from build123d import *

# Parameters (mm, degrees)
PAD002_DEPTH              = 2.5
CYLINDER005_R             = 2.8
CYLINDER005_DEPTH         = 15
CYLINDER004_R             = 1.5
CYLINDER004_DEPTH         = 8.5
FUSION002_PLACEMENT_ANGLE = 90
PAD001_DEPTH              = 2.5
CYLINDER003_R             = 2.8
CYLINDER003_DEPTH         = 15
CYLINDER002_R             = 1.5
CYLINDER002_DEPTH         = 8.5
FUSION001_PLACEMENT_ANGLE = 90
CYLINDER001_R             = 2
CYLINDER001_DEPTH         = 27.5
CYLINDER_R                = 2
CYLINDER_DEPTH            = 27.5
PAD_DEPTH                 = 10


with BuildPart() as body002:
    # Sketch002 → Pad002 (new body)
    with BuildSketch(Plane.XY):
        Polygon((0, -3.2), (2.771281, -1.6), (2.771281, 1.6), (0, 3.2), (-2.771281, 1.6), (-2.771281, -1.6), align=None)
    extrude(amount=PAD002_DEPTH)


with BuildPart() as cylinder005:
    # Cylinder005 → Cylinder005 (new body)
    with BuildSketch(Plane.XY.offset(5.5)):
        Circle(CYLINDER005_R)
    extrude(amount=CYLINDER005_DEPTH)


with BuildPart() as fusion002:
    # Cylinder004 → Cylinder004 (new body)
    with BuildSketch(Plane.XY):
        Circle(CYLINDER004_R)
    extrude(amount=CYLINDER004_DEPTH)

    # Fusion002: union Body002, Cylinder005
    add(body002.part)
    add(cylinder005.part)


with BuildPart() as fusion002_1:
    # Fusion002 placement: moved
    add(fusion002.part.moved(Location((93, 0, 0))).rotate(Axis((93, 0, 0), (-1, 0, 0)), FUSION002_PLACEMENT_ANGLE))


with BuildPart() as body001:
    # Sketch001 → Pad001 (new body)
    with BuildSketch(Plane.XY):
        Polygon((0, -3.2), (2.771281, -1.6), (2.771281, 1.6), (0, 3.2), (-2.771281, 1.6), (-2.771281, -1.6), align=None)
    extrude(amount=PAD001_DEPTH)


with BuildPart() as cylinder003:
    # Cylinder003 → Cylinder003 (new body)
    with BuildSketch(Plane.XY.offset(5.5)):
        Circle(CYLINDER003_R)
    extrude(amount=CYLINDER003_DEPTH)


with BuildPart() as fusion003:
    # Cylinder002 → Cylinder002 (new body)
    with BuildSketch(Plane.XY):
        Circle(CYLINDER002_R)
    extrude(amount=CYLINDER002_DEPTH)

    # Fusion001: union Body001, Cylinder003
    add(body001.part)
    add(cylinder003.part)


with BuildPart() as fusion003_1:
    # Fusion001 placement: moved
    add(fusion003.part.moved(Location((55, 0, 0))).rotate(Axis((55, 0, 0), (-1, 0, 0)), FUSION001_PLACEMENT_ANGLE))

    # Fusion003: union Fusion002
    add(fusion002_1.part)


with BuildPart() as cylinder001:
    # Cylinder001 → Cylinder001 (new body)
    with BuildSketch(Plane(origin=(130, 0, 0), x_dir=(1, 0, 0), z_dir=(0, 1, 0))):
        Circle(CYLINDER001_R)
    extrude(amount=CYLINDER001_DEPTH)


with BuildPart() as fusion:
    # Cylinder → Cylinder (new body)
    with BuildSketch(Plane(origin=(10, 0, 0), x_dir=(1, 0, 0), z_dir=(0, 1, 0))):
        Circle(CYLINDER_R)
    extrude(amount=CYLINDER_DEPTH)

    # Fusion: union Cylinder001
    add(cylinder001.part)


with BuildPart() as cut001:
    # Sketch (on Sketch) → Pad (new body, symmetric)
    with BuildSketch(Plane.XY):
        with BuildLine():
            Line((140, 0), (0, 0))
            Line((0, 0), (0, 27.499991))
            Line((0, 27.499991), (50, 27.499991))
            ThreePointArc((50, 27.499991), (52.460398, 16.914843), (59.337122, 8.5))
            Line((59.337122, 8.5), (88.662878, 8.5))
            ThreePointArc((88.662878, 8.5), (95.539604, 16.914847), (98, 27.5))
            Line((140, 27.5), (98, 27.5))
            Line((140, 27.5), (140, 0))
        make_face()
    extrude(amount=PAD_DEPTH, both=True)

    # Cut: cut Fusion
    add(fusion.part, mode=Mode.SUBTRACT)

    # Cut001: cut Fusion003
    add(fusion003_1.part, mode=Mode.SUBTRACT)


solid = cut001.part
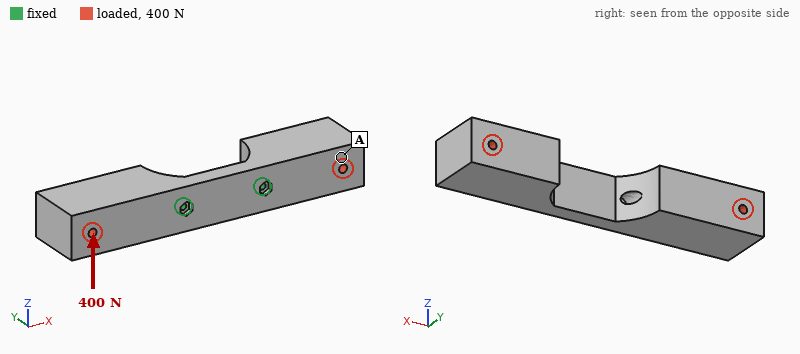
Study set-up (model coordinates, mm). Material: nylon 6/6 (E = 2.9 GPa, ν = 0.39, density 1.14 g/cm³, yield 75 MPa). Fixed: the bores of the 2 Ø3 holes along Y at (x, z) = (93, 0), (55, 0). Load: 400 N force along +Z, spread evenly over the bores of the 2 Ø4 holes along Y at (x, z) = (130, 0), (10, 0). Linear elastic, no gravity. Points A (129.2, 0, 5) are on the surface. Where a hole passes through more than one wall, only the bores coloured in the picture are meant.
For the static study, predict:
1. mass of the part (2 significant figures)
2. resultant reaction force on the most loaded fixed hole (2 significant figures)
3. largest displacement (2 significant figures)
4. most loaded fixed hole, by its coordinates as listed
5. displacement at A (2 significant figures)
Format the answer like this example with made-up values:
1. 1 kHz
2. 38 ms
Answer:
1. 68 g
2. 240 N
3. 1.4 mm
4. (55, 0)
5. 0.36 mm
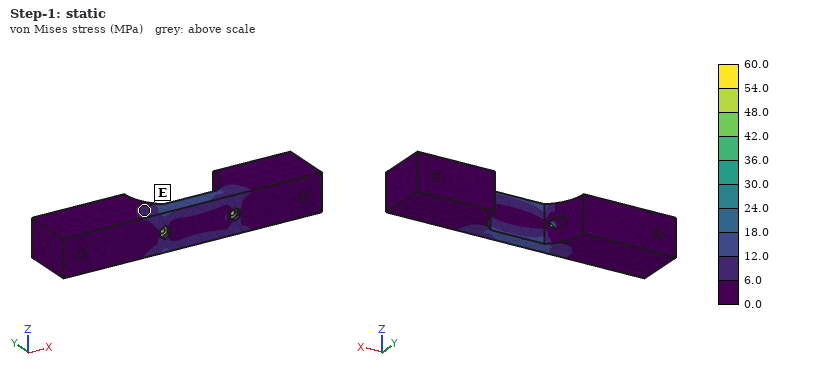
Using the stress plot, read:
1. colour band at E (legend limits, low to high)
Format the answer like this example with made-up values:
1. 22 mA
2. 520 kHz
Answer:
1. 6.0 to 12.0 MPa
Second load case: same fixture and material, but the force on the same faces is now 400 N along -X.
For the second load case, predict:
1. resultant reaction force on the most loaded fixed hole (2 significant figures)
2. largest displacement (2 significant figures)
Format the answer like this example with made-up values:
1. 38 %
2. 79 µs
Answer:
1. 220 N
2. 0.34 mm
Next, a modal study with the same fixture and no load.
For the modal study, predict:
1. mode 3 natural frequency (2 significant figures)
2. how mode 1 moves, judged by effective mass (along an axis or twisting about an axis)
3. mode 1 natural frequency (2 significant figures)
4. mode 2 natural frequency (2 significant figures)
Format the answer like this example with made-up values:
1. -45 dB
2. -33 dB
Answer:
1. 530 Hz
2. along Y
3. 380 Hz
4. 510 Hz
